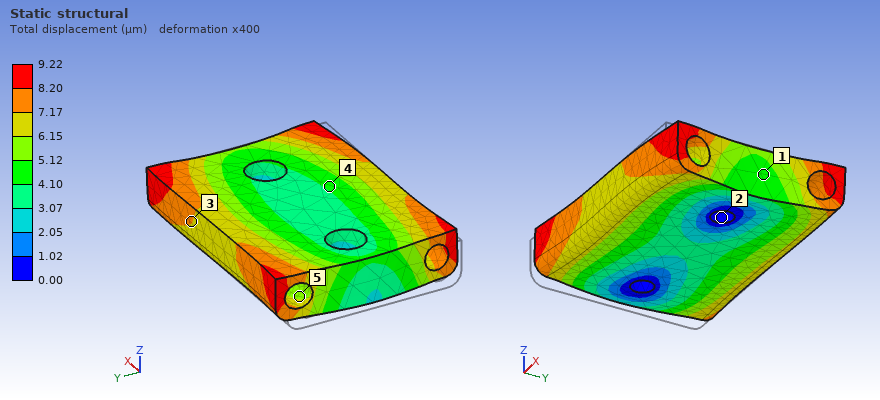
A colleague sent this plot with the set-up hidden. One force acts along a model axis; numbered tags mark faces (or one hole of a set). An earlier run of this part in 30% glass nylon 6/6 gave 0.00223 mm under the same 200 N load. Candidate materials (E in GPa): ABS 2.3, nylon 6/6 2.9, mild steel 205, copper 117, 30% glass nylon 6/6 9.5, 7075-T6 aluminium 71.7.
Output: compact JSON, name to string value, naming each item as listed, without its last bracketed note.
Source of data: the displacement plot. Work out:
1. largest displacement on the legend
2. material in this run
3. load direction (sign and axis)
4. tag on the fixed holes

{"largest displacement on the legend": "9.22 µm", "material in this run": "ABS", "load direction": "+X", "tag on the fixed holes": "2"}
